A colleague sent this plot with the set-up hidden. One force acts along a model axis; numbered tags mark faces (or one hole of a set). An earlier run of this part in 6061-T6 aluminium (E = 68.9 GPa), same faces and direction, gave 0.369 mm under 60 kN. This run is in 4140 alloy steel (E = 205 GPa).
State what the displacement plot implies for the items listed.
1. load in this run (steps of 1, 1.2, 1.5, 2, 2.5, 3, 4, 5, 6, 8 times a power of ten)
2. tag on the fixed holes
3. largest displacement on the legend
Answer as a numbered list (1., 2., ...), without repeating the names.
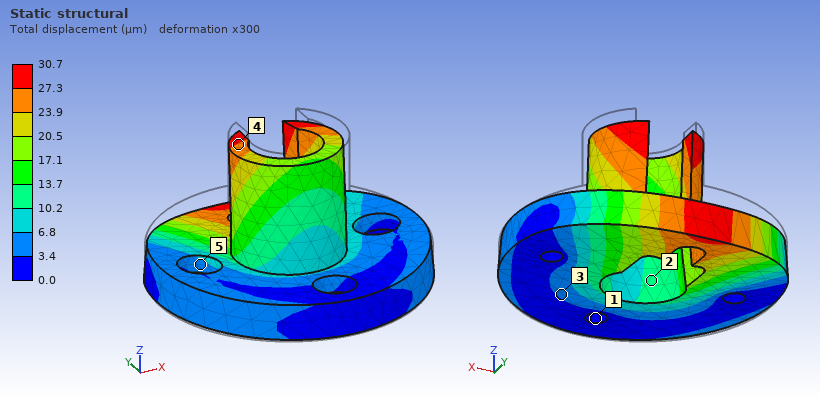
1. 15 kN
2. 1
3. 30.7 µm
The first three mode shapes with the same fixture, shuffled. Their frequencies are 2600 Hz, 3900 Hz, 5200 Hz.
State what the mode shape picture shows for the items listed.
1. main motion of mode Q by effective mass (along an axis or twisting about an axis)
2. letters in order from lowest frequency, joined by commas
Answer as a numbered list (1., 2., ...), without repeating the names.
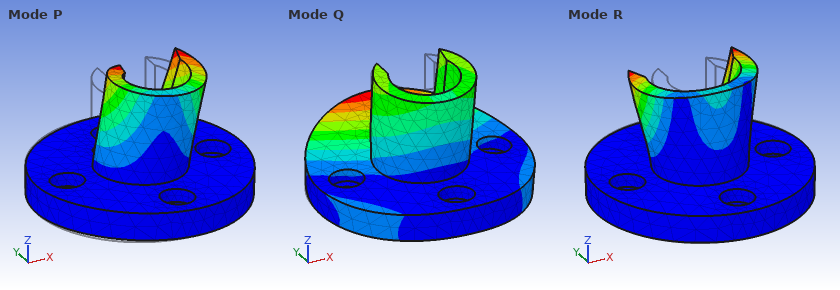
1. along Z
2. Q, P, R
